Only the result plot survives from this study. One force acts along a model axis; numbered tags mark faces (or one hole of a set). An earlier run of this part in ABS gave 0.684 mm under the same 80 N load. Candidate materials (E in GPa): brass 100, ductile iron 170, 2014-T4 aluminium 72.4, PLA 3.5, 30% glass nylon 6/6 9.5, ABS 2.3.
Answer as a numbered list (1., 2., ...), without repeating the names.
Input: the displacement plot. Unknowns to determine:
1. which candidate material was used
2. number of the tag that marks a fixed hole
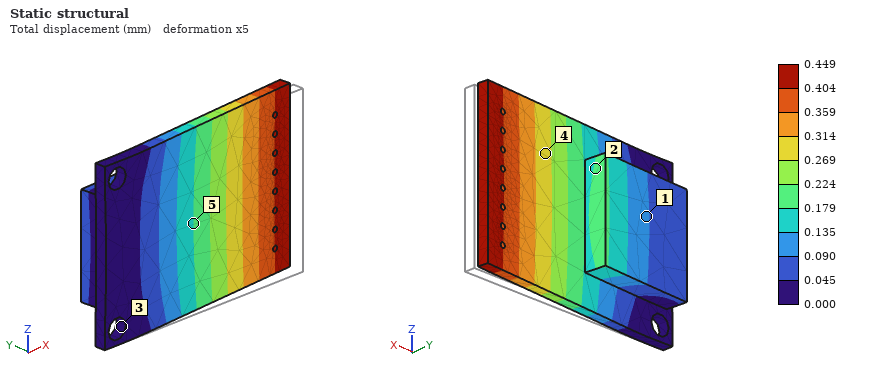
1. PLA
2. 3
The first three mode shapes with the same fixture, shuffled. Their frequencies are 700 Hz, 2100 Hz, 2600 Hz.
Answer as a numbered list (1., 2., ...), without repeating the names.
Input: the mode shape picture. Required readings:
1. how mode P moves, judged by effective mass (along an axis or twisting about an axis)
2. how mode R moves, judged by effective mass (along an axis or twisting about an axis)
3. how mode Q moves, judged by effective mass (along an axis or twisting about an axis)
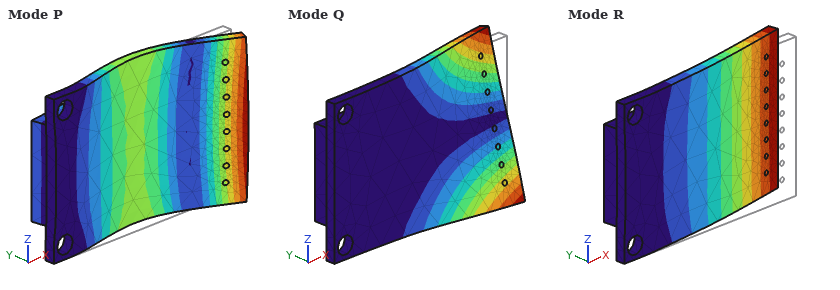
1. along Y
2. along Y
3. twisting about X
